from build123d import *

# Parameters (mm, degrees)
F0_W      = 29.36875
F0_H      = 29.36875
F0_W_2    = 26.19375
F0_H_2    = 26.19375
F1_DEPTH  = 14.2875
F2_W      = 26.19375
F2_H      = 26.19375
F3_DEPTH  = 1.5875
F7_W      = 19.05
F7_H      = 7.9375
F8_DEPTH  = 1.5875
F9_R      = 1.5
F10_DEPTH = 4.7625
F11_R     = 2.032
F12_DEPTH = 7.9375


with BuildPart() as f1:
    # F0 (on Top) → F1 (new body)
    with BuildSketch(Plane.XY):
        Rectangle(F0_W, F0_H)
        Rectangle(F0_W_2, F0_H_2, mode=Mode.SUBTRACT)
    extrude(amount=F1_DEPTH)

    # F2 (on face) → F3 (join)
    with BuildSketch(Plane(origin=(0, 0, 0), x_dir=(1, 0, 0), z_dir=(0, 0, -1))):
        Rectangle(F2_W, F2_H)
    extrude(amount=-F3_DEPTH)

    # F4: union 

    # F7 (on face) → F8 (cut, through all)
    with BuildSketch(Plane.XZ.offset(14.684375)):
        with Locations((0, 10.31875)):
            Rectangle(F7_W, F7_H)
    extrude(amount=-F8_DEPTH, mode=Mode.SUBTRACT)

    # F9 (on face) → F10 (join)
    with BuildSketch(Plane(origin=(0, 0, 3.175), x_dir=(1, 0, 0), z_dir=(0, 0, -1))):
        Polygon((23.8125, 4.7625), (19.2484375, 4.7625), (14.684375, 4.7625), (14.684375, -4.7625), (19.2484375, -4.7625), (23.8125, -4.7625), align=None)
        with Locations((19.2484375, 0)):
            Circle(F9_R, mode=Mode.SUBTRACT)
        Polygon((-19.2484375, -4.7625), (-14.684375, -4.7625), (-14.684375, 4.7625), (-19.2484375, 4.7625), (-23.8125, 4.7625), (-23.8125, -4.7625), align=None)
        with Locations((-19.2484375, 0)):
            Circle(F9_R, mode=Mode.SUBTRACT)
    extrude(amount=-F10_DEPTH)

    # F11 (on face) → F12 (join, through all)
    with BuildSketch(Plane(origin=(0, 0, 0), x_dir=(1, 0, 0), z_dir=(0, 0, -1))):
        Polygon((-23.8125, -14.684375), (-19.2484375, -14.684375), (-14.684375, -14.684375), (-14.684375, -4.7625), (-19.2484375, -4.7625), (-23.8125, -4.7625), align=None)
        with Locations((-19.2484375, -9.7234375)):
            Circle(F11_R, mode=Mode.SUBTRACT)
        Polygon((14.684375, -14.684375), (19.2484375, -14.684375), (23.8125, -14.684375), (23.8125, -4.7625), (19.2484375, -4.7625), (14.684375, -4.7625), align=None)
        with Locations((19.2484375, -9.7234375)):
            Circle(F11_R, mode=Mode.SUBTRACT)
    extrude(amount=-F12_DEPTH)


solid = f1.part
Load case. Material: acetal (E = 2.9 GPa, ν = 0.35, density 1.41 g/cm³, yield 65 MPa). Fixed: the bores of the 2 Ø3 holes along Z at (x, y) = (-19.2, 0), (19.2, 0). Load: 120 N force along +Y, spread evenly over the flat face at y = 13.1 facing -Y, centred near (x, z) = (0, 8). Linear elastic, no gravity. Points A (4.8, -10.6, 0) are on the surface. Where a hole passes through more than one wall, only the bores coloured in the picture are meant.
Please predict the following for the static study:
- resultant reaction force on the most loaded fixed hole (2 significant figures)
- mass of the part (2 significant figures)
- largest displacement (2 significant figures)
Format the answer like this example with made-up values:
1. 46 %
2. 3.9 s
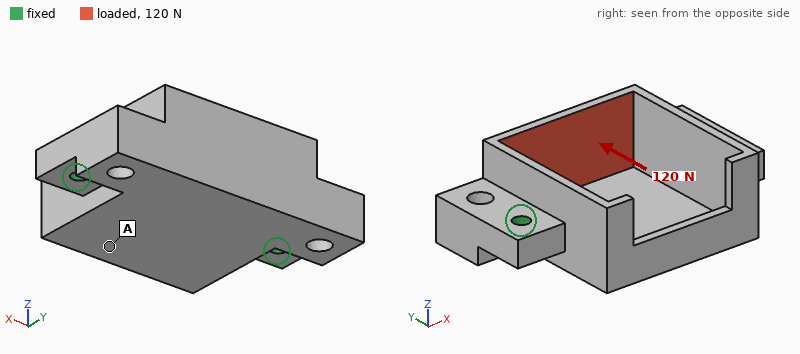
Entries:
1. 65 N
2. 7.6 g
3. 0.59 mm
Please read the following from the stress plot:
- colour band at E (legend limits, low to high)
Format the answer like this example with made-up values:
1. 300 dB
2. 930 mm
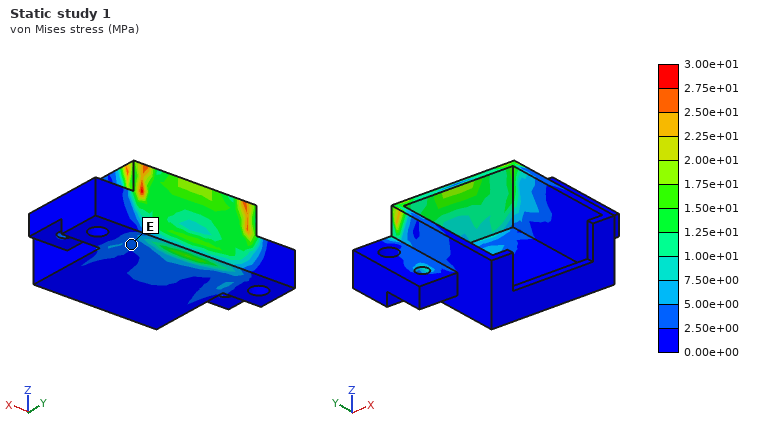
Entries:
1. 2.50e+00 to 5.00e+00 MPa
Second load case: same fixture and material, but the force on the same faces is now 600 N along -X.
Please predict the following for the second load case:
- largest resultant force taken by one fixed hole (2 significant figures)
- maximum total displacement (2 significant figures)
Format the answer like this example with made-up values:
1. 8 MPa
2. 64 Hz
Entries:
1. 330 N
2. 0.51 mm
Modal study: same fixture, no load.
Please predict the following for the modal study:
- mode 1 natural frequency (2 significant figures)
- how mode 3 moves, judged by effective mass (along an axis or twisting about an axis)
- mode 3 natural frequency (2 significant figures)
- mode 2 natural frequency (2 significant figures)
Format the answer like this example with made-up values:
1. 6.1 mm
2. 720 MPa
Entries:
1. 2300 Hz
2. along Z
3. 3400 Hz
4. 3200 Hz
